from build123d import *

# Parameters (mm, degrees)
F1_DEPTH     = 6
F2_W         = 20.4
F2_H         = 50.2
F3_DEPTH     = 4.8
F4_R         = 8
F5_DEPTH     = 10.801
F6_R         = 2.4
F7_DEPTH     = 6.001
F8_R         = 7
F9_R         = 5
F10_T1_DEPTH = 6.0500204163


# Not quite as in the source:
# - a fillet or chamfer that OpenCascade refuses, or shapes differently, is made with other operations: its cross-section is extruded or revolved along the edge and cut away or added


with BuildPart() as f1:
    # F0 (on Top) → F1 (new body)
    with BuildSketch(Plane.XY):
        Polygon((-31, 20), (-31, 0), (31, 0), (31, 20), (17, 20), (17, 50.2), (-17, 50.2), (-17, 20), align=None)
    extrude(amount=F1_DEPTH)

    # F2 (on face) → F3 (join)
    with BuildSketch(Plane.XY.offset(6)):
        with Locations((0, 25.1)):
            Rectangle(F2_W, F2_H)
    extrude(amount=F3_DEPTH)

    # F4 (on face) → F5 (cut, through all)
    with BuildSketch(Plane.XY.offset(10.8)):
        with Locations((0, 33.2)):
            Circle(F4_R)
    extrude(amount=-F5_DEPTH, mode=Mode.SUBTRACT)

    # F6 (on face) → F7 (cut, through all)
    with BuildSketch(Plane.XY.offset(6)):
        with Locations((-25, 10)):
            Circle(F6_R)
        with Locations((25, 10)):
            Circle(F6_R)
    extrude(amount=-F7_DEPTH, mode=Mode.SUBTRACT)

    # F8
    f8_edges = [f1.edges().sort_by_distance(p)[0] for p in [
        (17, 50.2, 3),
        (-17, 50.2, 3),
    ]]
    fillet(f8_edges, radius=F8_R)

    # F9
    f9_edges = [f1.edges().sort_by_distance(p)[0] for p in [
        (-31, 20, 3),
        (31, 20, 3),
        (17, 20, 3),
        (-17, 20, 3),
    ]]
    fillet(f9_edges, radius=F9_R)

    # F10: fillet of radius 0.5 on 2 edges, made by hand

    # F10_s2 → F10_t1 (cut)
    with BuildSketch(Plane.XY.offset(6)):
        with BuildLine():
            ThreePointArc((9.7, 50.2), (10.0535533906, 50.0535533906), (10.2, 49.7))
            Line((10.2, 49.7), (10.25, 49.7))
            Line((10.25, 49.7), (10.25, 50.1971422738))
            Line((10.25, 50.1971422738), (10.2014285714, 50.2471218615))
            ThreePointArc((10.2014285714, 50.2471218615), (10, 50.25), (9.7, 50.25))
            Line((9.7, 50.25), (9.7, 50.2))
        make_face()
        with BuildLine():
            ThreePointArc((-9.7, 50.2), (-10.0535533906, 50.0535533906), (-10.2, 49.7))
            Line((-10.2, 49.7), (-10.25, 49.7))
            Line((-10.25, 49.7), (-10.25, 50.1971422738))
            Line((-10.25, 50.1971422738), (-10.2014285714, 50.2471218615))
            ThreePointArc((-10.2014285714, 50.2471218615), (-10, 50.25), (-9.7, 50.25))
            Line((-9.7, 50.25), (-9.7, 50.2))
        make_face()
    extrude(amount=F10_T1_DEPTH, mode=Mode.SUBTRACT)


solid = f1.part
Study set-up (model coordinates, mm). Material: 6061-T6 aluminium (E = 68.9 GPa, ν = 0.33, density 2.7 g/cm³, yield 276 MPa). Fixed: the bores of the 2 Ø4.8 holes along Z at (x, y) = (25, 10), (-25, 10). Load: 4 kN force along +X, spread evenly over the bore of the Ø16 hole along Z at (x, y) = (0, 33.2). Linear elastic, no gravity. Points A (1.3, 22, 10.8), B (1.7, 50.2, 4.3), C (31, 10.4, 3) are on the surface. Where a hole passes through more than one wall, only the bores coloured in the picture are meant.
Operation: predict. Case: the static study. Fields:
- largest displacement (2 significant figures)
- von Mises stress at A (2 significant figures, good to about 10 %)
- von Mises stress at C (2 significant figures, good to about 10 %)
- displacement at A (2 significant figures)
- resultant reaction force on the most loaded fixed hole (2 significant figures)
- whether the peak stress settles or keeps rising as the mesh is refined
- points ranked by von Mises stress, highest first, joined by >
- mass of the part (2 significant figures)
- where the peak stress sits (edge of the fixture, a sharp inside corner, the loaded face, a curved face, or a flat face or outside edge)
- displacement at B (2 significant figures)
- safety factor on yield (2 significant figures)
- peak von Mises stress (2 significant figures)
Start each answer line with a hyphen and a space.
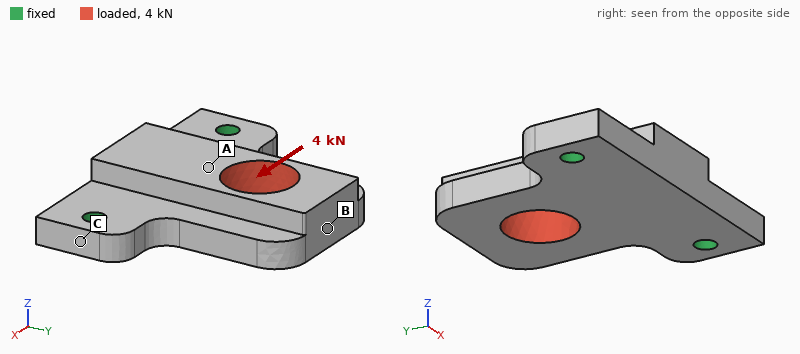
- 52 µm
- 34 MPa
- 19 MPa
- 12 µm
- 2.8 kN
- settles
- A > C > B
- 43 g
- a curved face
- 48 µm
- 2.2
- 130 MPa
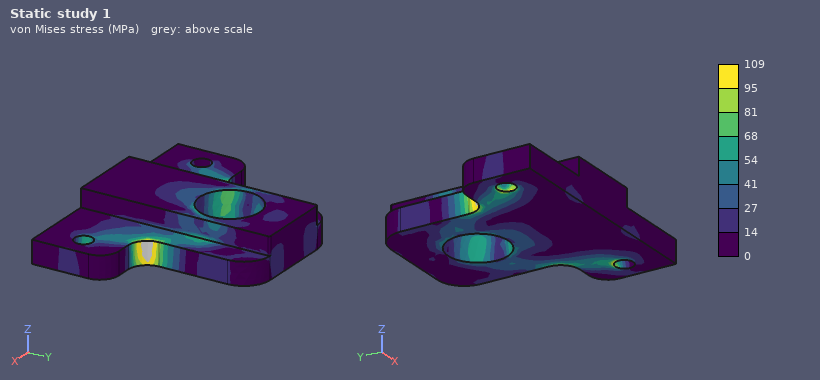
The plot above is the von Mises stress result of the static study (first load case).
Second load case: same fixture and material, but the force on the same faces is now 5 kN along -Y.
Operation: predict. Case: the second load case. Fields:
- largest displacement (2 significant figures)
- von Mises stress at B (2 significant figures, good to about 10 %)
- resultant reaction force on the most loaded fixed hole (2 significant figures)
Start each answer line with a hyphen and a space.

- 0.14 mm
- 15 MPa
- 2.6 kN
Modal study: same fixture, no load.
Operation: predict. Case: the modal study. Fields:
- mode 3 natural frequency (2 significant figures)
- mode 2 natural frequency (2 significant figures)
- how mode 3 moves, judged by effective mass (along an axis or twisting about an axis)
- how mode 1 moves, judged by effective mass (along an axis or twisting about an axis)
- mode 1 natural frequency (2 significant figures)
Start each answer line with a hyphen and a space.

- 11 kHz
- 9400 Hz
- along X
- along Z
- 2700 Hz
